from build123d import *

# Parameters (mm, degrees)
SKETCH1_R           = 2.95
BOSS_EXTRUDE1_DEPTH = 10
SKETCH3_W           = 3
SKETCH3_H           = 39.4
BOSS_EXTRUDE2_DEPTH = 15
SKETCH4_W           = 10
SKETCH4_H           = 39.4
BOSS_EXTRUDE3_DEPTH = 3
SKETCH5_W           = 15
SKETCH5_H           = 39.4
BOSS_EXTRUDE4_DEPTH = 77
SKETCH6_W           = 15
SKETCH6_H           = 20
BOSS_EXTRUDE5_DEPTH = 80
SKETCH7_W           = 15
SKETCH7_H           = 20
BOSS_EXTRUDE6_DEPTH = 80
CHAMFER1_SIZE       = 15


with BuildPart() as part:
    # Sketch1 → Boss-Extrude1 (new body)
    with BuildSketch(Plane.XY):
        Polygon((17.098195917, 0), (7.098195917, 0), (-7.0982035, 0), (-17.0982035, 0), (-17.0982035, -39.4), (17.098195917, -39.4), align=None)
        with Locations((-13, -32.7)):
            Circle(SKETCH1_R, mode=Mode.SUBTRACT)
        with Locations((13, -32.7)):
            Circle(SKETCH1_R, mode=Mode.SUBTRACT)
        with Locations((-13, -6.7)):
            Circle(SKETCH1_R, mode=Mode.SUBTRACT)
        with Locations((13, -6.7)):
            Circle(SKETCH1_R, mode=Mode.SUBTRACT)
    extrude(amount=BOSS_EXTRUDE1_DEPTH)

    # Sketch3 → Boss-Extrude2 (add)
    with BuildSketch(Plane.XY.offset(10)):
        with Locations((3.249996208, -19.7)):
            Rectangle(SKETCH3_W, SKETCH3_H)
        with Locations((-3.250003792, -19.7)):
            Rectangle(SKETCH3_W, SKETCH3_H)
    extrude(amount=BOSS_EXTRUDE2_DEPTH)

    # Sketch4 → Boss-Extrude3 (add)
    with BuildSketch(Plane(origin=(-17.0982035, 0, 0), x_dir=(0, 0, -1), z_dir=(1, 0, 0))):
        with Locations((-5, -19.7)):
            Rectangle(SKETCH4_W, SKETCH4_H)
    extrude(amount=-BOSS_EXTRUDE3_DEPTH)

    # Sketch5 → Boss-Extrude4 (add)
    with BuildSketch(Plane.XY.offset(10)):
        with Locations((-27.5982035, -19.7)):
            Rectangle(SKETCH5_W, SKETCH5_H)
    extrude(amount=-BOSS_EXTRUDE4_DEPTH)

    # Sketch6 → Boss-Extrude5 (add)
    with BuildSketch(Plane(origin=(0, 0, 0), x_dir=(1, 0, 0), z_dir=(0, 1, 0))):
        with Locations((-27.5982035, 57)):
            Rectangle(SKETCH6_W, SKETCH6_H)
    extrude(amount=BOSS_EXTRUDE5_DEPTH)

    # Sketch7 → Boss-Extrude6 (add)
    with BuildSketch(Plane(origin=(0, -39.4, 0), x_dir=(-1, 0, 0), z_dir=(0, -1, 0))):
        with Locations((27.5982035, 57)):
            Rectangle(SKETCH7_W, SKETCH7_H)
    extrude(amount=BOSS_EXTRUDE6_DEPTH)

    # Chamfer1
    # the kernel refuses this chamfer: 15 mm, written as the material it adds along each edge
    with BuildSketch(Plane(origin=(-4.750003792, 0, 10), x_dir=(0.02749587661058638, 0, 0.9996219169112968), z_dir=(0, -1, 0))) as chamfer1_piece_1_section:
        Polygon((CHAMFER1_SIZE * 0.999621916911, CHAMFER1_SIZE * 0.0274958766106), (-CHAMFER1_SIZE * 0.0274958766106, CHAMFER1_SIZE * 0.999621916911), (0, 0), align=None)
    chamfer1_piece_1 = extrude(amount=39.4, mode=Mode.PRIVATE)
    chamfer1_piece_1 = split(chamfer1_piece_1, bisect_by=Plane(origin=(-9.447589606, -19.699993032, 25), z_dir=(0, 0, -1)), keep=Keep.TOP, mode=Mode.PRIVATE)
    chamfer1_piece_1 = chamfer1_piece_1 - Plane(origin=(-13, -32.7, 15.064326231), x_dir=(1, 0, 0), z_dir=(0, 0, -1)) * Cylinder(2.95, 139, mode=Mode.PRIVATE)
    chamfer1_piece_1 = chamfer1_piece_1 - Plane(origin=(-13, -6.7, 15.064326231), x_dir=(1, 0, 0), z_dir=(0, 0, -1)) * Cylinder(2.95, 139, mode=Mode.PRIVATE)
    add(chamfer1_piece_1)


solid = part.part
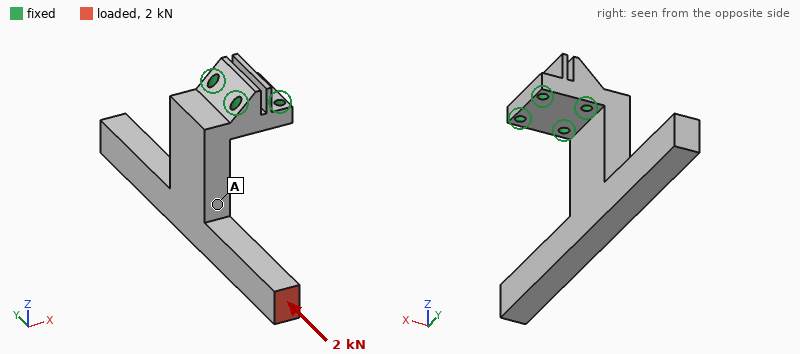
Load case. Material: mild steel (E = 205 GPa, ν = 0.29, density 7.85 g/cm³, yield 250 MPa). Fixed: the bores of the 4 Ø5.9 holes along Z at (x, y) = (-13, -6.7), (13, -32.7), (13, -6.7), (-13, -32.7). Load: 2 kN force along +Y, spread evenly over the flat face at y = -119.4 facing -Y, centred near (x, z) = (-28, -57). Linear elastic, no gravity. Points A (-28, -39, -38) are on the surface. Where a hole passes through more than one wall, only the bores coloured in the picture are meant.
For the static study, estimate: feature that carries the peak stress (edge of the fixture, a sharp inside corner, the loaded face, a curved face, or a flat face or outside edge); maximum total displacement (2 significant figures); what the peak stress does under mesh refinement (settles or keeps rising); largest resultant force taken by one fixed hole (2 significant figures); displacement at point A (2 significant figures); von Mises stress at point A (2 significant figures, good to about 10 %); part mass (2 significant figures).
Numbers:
edge of the fixture
78 µm
keeps rising
4.3 kN
25 µm
12 MPa
900 g
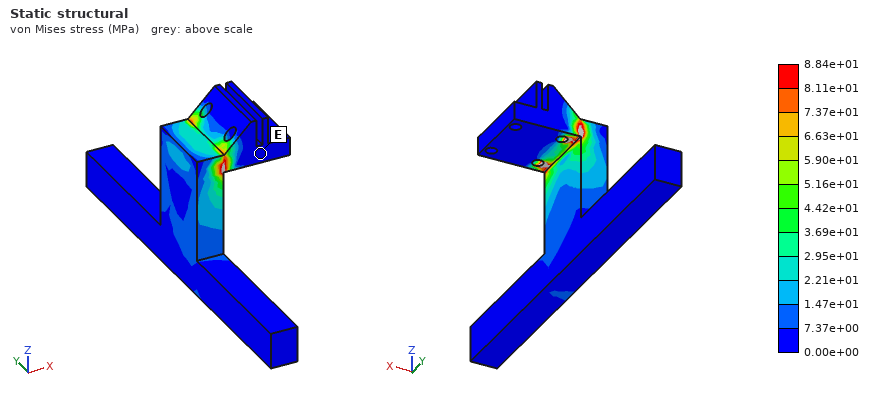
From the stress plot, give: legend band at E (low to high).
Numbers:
0.00e+00 to 7.37e+00 MPa
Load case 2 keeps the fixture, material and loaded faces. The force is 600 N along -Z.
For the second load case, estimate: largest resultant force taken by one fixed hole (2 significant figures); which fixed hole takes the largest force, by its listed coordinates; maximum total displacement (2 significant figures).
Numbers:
2.3 kN
(-13, -32.7)
0.12 mm
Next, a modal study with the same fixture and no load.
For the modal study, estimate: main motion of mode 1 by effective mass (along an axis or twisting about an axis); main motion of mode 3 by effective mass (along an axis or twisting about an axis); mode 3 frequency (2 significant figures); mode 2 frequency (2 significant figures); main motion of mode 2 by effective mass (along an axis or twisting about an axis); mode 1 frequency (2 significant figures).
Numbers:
along X
along Y
1100 Hz
770 Hz
twisting about Z
700 Hz
